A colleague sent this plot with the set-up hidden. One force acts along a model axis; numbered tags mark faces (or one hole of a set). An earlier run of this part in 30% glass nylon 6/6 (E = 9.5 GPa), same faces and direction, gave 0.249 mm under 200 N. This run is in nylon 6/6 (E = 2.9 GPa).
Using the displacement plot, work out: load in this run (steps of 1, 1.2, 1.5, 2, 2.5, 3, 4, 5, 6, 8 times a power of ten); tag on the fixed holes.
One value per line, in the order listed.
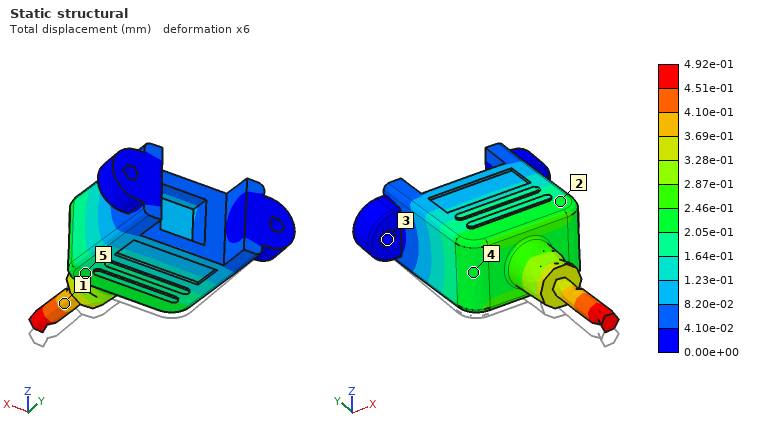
120 N
3
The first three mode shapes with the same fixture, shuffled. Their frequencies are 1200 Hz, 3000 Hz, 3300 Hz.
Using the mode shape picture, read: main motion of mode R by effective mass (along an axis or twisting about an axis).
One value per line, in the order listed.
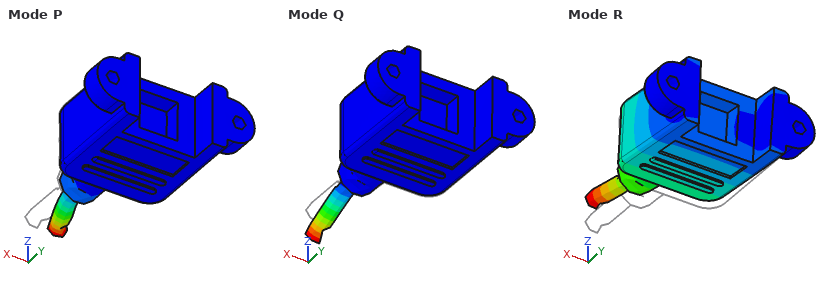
along Z
